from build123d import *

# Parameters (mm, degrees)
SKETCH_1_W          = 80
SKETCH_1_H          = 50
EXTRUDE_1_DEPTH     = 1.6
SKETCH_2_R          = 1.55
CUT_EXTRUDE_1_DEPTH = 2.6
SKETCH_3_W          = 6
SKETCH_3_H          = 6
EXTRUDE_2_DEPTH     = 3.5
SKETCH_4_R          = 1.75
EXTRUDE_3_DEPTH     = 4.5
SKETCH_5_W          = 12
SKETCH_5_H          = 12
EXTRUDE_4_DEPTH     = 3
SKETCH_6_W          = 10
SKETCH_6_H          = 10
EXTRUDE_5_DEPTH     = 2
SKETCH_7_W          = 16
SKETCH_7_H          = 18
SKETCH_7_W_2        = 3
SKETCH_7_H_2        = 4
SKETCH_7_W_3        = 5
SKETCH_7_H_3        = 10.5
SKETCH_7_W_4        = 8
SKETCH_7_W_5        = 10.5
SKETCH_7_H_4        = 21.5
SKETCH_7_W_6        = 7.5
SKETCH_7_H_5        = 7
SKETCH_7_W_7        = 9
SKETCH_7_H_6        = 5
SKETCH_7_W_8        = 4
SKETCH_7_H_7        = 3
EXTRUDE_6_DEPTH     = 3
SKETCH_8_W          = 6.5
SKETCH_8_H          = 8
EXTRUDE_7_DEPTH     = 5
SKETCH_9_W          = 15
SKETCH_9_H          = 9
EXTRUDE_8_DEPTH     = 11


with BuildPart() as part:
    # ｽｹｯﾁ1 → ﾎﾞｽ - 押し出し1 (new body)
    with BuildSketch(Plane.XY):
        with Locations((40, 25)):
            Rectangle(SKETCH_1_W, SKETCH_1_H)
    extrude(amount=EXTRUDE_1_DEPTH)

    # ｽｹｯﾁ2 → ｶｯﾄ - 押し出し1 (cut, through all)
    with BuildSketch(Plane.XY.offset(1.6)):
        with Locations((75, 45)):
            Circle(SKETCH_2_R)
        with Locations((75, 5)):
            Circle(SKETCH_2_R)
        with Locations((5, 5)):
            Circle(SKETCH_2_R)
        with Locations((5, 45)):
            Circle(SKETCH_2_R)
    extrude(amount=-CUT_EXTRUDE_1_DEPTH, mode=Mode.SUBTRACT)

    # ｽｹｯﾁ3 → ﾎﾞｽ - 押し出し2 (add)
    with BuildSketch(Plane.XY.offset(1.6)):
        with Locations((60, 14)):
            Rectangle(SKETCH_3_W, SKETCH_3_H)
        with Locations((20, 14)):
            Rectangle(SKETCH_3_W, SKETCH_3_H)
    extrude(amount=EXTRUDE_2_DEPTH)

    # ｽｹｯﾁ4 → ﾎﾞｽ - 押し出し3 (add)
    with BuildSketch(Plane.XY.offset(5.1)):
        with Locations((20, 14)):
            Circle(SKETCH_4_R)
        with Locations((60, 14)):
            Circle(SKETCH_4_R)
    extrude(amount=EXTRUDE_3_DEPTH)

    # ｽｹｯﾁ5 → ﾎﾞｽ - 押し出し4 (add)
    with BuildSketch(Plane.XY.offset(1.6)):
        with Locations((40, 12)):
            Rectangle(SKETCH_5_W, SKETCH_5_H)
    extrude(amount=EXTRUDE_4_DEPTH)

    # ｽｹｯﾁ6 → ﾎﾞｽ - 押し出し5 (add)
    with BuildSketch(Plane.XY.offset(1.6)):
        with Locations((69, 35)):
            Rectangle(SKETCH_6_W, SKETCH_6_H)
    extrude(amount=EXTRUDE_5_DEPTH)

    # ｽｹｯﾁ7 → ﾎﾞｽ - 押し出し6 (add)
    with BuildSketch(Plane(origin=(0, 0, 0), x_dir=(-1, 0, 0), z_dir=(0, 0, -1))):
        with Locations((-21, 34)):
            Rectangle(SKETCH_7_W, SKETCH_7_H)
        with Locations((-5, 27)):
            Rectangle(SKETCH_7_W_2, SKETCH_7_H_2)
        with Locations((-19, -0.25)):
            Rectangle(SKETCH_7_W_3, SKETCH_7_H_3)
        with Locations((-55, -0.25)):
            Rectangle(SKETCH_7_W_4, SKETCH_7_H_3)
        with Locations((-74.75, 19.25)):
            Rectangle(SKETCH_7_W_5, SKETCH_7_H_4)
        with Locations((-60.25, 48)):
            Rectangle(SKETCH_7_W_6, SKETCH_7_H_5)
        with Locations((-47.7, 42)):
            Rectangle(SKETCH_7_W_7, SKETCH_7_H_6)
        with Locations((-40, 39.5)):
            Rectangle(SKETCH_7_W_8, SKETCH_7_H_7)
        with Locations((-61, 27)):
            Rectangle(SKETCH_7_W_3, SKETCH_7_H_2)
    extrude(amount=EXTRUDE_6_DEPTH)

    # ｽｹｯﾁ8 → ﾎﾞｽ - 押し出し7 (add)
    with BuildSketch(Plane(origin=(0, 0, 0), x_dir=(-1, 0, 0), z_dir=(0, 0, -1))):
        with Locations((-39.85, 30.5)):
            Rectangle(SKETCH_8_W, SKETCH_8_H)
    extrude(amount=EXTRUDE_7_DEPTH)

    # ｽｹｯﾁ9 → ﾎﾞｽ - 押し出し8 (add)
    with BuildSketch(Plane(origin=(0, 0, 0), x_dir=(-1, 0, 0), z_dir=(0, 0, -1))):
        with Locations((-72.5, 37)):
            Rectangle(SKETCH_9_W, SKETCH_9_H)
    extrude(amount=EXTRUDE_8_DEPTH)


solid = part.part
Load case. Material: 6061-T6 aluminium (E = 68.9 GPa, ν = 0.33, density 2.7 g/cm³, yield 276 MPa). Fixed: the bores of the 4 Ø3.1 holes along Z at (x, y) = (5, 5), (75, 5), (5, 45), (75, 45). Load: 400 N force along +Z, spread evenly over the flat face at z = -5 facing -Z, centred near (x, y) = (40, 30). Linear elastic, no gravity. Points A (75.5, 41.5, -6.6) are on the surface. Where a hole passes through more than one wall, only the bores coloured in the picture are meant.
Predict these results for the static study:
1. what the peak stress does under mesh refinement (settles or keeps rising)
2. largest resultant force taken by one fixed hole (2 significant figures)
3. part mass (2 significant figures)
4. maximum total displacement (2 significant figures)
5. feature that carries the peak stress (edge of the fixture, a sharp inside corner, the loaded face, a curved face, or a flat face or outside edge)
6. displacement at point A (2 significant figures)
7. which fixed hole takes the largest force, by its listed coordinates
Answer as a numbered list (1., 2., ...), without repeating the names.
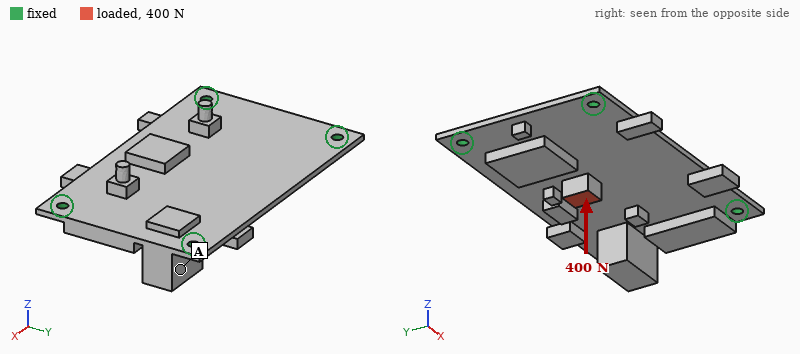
1. keeps rising
2. 150 N
3. 31 g
4. 0.49 mm
5. edge of the fixture
6. 0.075 mm
7. (75, 45)
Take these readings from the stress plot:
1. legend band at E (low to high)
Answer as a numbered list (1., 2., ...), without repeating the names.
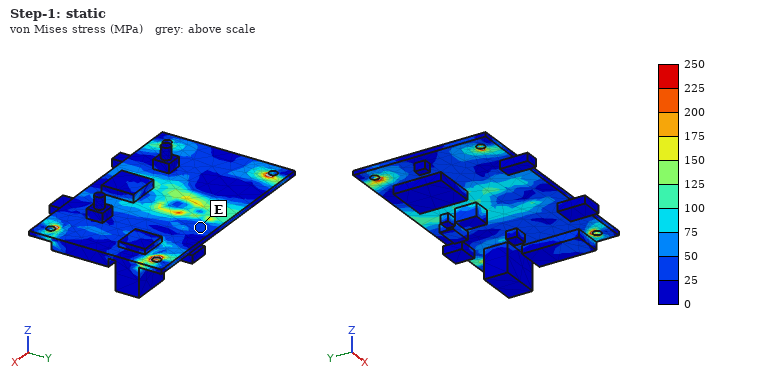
1. 25 to 50 MPa
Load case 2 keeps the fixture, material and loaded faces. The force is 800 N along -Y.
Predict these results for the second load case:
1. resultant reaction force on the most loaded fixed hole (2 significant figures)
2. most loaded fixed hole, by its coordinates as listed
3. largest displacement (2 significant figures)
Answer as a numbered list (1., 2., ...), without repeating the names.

1. 330 N
2. (5, 45)
3. 0.20 mm
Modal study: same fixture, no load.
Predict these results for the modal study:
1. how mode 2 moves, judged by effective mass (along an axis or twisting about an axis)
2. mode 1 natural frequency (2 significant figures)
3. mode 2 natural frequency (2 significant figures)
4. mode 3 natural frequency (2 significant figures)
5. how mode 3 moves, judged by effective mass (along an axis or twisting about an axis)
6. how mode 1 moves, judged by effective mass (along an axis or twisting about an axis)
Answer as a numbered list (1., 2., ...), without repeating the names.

1. twisting about X
2. 1500 Hz
3. 2600 Hz
4. 3800 Hz
5. twisting about Y
6. along Z
